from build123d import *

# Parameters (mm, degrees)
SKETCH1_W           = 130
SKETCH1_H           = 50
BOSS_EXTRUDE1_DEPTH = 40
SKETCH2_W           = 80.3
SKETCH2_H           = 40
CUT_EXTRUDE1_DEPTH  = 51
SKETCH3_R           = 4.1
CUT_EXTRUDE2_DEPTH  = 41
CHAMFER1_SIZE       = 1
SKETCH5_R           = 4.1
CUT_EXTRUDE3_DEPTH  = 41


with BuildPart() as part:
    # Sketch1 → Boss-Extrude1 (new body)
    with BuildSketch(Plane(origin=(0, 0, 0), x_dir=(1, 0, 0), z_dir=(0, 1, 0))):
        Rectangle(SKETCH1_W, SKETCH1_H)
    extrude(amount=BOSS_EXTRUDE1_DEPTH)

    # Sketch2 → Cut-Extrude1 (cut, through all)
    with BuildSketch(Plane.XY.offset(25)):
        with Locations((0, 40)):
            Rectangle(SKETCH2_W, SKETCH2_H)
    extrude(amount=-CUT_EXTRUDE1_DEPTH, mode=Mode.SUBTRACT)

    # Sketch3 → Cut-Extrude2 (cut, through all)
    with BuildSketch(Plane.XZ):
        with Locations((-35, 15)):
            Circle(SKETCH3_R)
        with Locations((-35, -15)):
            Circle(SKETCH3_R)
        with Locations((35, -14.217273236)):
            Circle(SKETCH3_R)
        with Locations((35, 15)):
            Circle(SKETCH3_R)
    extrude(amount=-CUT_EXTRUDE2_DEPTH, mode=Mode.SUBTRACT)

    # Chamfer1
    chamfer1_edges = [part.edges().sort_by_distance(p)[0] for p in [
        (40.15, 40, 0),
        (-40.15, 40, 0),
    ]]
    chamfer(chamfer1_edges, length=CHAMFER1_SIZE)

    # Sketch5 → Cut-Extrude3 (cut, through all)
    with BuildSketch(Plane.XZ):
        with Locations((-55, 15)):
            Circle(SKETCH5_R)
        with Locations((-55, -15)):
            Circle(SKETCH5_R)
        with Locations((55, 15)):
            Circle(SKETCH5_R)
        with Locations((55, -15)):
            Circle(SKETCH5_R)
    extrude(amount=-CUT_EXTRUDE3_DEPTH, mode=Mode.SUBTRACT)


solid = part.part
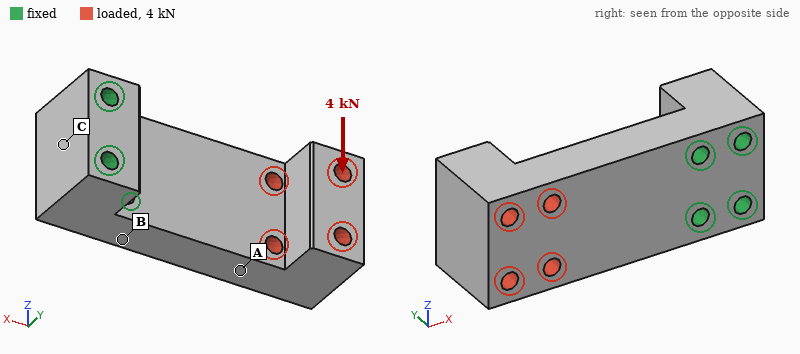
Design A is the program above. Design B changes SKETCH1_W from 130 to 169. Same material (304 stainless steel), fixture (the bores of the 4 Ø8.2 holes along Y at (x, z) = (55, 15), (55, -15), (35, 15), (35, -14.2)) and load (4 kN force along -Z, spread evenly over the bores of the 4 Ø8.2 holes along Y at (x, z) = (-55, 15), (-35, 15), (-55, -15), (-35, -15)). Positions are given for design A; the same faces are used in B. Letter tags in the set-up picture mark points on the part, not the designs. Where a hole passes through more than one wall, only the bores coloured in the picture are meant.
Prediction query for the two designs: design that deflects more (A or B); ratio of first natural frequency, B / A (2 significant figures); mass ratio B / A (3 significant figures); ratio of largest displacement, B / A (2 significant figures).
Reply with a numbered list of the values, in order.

1. B
2. 0.65
3. 1.47
4. 1.2
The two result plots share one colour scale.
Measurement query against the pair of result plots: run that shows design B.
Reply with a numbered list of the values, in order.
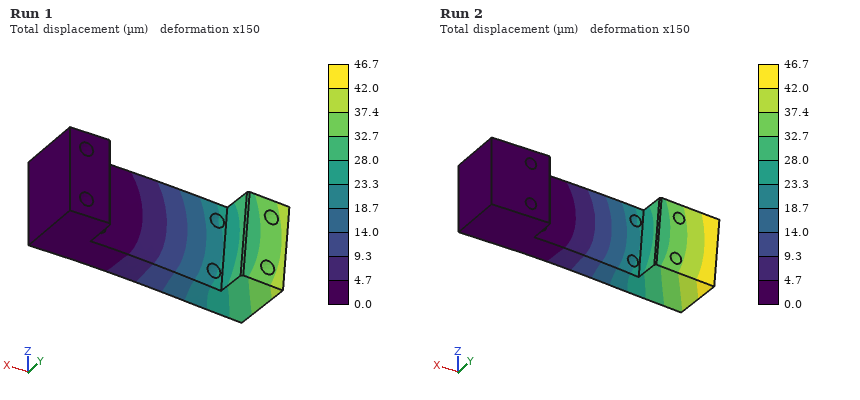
1. Run 2
